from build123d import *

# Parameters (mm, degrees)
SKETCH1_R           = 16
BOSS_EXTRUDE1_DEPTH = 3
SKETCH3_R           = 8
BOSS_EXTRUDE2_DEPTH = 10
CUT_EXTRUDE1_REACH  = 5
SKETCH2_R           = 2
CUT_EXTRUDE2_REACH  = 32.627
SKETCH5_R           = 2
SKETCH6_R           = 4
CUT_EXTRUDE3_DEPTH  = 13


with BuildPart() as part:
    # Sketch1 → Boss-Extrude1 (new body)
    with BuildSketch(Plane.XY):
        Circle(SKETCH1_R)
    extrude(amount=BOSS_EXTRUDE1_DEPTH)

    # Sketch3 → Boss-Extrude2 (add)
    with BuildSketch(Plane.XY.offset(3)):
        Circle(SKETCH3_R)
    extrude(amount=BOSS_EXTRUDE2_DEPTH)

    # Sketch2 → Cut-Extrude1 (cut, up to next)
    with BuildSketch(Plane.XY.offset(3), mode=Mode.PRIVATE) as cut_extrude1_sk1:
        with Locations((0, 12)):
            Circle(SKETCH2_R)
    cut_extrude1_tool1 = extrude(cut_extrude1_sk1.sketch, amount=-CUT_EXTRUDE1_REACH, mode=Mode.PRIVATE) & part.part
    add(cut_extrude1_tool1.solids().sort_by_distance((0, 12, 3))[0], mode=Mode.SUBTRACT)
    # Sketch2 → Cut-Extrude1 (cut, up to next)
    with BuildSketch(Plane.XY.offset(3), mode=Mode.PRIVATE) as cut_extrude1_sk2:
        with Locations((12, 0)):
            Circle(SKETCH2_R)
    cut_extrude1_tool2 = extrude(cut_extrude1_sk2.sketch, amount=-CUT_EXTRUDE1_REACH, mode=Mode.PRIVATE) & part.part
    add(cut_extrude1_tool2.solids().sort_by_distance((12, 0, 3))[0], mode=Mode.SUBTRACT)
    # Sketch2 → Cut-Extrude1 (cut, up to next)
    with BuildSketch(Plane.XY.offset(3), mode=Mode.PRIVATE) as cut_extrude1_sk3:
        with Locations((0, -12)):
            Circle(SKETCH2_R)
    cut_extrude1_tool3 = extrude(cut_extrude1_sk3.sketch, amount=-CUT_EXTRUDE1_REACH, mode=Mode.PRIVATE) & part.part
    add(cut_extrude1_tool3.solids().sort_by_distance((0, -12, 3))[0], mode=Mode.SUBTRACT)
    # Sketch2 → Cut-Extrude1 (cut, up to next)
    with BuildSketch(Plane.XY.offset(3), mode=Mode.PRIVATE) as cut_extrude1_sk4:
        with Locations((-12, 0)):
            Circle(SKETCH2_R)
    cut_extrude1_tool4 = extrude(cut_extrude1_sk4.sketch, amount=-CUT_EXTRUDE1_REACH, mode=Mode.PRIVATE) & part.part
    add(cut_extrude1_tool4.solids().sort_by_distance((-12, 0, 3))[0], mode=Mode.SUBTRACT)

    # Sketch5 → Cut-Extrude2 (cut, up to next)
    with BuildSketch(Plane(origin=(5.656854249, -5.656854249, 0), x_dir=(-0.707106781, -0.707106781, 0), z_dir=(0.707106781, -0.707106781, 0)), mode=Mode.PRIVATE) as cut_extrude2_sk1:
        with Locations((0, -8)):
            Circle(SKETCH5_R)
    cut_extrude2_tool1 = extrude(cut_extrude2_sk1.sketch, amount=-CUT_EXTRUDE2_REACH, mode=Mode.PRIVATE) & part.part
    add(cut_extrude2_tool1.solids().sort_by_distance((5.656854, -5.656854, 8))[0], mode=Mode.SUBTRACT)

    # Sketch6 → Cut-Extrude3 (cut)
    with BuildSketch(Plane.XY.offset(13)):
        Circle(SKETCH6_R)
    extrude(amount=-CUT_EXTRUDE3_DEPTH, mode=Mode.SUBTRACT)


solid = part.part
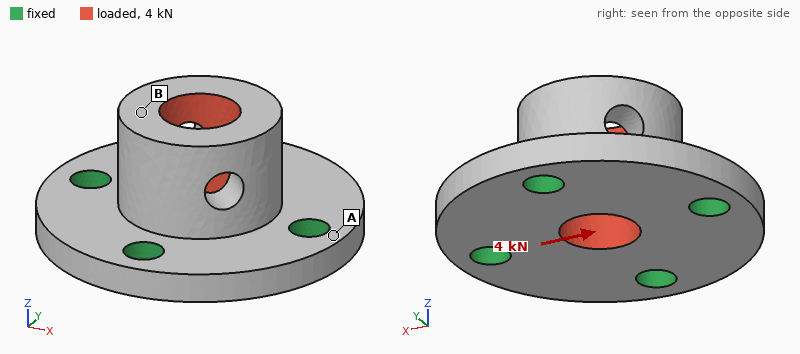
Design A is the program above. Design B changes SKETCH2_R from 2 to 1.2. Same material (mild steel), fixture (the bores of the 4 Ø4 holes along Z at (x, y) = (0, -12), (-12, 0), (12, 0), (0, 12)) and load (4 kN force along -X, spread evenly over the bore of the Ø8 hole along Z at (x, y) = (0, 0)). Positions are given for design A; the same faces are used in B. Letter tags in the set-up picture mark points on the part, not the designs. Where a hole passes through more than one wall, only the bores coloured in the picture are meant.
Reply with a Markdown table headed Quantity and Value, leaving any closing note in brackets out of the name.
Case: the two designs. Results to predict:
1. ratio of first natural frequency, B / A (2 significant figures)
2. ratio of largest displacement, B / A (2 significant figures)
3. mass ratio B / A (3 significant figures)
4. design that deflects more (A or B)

| Quantity | Value |
|---|---|
| ratio of first natural frequency, B / A | 0.87 |
| ratio of largest displacement, B / A | 1.2 |
| mass ratio B / A | 1.03 |
| design that deflects more | B |
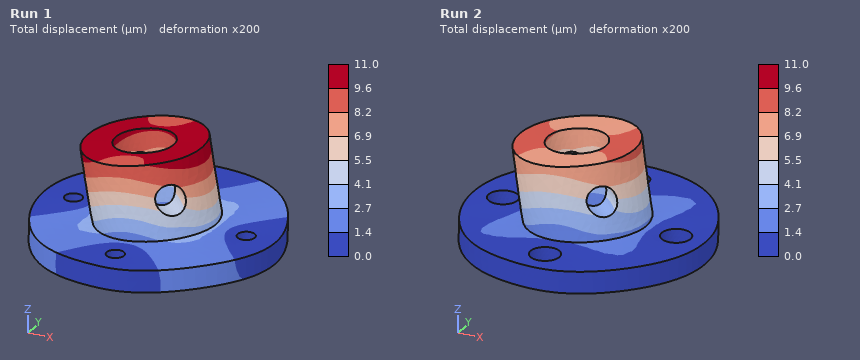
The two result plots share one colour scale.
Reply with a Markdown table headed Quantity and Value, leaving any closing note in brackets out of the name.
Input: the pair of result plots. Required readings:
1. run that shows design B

| Quantity | Value |
|---|---|
| run that shows design B | Run 1 |
